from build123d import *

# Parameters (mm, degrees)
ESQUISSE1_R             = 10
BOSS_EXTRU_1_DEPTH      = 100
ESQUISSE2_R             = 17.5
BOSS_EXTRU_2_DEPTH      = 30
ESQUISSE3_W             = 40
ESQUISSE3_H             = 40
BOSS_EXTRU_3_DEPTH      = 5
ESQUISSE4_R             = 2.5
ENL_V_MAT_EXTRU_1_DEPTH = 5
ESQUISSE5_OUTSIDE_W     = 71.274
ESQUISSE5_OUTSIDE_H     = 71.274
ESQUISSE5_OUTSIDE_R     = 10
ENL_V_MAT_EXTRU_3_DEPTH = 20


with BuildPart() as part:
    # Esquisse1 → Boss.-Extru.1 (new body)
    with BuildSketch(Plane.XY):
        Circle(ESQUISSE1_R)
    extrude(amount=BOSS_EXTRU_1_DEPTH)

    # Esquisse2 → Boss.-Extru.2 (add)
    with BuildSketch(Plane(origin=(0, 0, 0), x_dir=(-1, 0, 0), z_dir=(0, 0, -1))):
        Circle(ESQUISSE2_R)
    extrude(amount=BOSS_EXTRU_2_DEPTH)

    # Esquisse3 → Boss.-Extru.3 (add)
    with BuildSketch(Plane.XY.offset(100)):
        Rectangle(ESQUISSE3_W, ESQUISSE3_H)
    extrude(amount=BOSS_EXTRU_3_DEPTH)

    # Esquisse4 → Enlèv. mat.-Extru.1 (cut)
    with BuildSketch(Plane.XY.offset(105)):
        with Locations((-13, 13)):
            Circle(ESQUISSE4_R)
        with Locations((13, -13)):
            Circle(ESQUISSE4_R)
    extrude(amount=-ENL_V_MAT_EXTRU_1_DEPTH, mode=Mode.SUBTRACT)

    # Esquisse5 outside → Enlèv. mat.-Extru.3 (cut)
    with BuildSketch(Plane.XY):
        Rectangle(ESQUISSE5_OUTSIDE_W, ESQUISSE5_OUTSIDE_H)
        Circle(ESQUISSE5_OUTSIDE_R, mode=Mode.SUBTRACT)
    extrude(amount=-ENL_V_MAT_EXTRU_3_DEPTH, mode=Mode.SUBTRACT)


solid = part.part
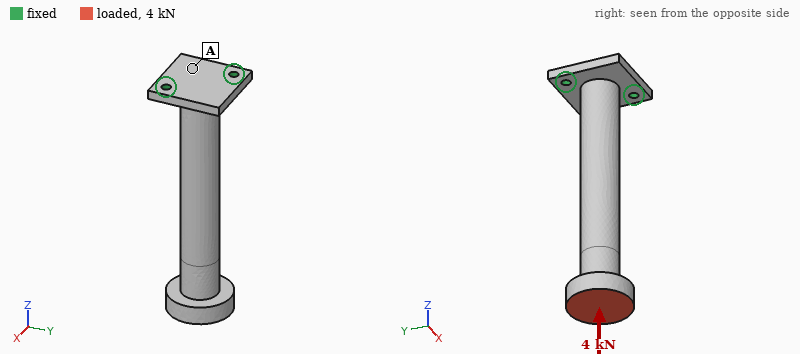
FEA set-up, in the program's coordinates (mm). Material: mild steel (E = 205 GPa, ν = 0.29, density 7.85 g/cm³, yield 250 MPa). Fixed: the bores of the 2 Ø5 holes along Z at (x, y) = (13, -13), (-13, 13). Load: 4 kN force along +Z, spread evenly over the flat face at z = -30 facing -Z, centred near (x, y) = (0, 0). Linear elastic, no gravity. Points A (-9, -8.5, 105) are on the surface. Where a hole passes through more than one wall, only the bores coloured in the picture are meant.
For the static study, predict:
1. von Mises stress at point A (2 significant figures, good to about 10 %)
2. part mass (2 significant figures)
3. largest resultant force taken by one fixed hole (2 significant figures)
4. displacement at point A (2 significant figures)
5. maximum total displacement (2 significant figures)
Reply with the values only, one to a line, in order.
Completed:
22 MPa
430 g
2.1 kN
9.5 µm
17 µm
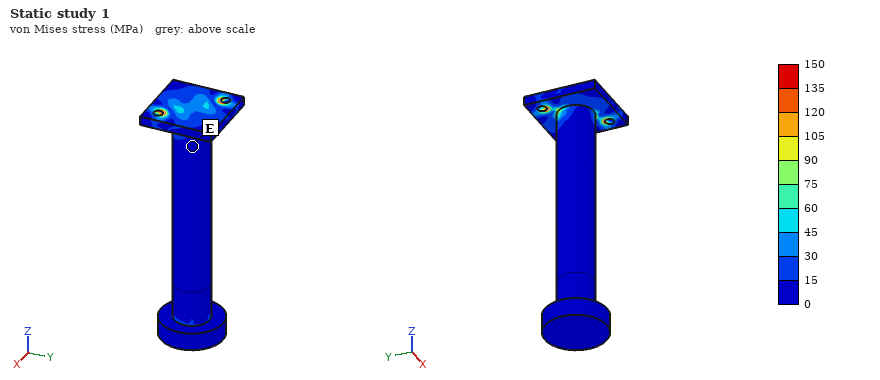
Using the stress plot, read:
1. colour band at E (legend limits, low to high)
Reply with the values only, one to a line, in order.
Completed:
0 to 15 MPa
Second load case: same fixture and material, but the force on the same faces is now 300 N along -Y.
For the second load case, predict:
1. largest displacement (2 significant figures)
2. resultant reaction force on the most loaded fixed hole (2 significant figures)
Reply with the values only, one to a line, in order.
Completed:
0.36 mm
1000 N
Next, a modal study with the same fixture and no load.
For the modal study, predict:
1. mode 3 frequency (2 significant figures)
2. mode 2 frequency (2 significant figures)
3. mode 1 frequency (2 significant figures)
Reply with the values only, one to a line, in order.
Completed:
3100 Hz
540 Hz
330 Hz
